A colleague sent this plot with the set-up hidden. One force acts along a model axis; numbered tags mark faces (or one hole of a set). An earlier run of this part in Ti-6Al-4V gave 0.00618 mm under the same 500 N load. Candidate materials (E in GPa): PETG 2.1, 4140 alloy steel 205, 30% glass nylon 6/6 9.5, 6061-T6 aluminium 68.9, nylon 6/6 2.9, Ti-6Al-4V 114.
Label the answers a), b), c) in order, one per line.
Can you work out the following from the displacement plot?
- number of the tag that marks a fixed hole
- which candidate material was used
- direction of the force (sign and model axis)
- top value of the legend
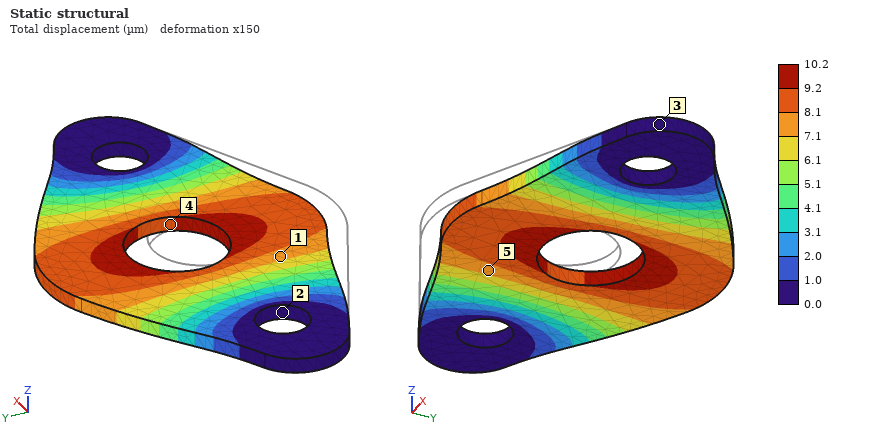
a) 2
b) 6061-T6 aluminium
c) +Y
d) 10.2 µm
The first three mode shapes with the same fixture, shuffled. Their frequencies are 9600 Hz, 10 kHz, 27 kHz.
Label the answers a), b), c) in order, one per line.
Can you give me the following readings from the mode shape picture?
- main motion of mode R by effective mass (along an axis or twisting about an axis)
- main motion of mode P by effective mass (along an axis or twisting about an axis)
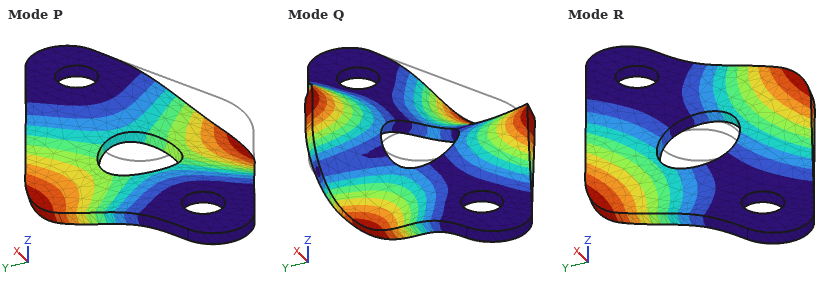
a) twisting about X
b) along Z
